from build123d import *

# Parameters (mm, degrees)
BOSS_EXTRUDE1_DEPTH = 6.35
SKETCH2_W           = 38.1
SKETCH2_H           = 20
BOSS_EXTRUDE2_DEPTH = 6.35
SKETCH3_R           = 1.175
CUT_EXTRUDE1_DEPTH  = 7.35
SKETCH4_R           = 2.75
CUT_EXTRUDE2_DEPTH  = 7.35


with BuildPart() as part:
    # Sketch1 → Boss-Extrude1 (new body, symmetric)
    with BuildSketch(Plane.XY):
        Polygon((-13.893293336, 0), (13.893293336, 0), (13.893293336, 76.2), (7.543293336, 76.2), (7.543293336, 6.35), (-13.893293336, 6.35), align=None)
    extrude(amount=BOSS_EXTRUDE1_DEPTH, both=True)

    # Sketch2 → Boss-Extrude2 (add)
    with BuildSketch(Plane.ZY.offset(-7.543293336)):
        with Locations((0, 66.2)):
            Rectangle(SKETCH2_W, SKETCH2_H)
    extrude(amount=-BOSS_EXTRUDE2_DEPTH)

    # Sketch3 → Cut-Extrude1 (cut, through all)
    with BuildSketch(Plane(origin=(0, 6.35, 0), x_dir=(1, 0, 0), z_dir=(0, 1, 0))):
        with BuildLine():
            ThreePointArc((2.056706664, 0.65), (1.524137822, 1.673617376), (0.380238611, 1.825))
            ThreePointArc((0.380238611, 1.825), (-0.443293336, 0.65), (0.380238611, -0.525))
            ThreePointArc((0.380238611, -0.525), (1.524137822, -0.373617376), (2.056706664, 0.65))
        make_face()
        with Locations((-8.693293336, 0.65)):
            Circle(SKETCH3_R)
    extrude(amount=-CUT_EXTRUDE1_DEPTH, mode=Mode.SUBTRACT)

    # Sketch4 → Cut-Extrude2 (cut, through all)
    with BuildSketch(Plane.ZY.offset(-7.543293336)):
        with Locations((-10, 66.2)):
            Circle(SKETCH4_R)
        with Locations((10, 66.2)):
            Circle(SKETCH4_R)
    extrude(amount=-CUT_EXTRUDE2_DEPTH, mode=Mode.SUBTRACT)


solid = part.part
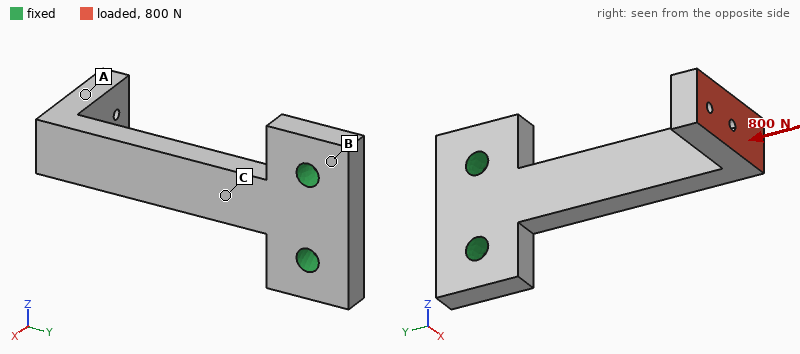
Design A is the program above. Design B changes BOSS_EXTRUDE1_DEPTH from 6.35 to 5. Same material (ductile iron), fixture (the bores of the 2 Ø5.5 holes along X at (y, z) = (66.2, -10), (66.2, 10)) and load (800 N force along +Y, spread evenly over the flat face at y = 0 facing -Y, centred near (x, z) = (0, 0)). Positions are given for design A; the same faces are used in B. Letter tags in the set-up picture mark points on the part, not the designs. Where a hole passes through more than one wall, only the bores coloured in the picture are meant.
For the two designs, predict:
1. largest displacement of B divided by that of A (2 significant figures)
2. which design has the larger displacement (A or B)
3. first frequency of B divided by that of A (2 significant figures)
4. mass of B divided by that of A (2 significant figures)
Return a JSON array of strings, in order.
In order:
["1.3", "B", "1.0", "0.88"]
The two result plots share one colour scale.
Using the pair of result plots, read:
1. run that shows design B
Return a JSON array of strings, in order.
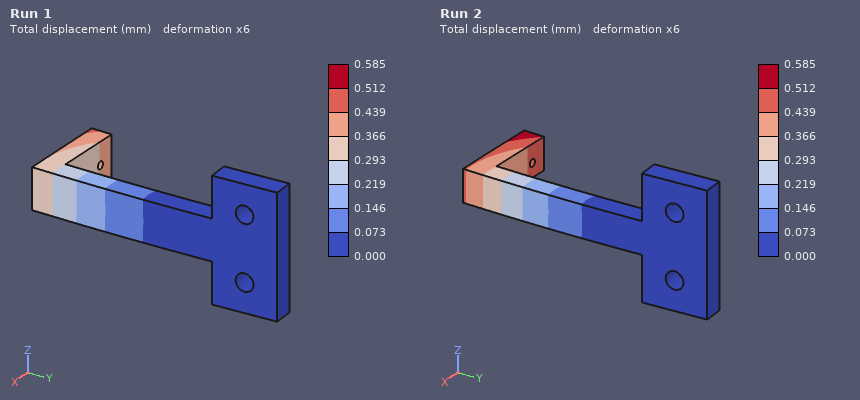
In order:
["Run 2"]
